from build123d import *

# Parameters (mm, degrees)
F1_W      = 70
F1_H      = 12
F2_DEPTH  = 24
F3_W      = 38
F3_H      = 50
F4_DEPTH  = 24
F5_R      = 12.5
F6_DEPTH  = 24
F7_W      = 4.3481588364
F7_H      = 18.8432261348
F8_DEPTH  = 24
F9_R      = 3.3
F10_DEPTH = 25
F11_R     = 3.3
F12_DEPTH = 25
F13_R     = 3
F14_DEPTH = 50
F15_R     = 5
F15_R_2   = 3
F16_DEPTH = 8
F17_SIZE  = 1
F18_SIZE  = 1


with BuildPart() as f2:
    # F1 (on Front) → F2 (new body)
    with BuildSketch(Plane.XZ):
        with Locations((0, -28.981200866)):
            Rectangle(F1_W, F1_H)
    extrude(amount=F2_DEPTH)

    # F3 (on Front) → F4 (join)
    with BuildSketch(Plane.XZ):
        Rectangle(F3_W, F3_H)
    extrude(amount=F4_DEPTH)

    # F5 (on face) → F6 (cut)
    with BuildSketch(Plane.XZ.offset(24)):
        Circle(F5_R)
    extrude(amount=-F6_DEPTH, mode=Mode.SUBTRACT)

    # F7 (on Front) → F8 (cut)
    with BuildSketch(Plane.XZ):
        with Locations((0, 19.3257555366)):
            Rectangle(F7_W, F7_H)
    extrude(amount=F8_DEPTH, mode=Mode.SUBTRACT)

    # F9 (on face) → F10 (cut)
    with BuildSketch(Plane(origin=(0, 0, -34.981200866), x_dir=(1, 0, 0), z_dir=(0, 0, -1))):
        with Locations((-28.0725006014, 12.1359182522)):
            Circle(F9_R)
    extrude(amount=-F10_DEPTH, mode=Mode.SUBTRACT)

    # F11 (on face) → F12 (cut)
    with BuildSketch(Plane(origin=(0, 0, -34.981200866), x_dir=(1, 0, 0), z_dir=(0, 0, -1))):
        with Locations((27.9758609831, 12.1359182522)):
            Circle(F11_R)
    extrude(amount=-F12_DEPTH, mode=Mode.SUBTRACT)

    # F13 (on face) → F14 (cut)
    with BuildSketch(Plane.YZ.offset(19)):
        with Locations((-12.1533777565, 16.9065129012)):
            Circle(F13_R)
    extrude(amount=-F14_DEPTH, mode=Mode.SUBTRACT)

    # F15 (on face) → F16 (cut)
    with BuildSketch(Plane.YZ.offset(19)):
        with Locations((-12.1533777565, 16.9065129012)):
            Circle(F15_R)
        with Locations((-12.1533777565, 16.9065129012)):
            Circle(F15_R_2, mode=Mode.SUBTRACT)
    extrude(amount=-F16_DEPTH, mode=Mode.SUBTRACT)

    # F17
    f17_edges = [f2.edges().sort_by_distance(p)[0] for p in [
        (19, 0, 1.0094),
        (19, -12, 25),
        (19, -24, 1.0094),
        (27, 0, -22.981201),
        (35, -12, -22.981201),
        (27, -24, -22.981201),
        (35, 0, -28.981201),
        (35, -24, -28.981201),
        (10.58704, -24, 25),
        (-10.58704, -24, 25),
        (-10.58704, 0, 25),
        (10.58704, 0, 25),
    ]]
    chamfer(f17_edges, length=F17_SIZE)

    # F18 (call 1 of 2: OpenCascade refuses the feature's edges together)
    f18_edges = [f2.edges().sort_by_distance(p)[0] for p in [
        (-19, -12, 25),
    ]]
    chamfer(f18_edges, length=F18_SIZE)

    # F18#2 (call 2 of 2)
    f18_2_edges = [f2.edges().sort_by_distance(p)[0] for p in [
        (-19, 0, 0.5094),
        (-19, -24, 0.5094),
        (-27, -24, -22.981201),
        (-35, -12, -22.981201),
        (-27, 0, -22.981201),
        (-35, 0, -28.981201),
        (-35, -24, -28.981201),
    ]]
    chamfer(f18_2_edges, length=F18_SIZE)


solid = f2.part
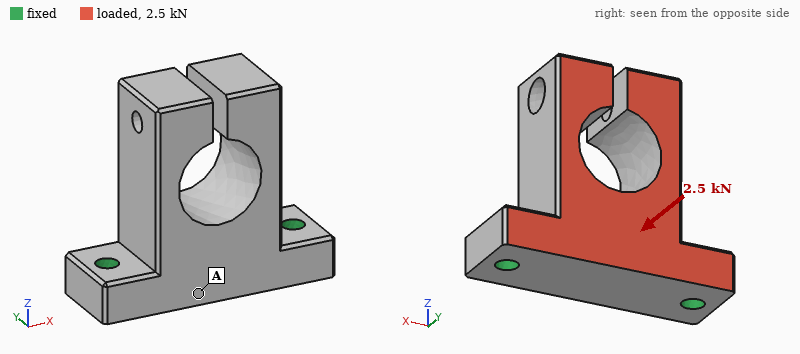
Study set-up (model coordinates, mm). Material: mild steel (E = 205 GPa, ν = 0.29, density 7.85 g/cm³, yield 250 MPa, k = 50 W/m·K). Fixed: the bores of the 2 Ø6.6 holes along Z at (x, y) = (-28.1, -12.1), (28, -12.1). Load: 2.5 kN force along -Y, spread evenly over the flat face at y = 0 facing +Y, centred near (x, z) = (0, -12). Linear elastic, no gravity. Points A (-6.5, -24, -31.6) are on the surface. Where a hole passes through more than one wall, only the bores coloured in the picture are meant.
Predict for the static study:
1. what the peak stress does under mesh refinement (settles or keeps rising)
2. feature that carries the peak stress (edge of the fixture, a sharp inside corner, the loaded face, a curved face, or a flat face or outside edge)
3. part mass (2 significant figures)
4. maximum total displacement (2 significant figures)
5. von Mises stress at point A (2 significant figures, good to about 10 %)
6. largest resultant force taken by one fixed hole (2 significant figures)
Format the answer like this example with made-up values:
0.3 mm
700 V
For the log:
keeps rising
edge of the fixture
380 g
27 µm
8.3 MPa
1.3 kN
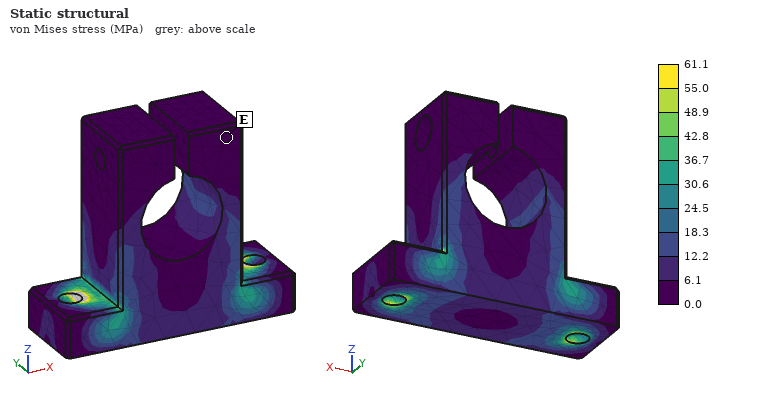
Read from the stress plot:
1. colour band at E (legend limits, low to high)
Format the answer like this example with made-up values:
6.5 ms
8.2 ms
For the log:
0.0 to 6.1 MPa
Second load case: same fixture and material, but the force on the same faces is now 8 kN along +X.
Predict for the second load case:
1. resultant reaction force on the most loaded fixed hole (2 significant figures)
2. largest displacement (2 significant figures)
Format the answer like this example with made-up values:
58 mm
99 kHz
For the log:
5.2 kN
0.10 mm
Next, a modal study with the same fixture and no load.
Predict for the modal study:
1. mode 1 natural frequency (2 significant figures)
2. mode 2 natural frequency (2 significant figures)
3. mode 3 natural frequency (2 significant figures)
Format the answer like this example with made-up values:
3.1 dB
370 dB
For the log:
2900 Hz
3000 Hz
3000 Hz
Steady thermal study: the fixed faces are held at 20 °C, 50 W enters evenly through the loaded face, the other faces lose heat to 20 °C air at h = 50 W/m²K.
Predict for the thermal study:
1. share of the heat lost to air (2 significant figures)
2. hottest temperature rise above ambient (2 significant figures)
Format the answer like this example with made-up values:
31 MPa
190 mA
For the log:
23 %
37 K
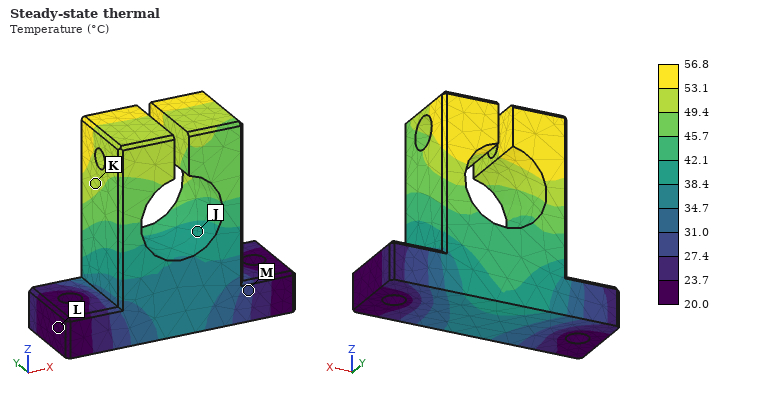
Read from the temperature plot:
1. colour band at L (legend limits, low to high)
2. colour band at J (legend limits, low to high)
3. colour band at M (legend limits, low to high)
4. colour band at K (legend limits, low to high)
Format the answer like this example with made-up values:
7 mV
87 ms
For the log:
20.0 to 23.7 °C
38.4 to 42.1 °C
27.4 to 31.0 °C
49.4 to 53.1 °C
